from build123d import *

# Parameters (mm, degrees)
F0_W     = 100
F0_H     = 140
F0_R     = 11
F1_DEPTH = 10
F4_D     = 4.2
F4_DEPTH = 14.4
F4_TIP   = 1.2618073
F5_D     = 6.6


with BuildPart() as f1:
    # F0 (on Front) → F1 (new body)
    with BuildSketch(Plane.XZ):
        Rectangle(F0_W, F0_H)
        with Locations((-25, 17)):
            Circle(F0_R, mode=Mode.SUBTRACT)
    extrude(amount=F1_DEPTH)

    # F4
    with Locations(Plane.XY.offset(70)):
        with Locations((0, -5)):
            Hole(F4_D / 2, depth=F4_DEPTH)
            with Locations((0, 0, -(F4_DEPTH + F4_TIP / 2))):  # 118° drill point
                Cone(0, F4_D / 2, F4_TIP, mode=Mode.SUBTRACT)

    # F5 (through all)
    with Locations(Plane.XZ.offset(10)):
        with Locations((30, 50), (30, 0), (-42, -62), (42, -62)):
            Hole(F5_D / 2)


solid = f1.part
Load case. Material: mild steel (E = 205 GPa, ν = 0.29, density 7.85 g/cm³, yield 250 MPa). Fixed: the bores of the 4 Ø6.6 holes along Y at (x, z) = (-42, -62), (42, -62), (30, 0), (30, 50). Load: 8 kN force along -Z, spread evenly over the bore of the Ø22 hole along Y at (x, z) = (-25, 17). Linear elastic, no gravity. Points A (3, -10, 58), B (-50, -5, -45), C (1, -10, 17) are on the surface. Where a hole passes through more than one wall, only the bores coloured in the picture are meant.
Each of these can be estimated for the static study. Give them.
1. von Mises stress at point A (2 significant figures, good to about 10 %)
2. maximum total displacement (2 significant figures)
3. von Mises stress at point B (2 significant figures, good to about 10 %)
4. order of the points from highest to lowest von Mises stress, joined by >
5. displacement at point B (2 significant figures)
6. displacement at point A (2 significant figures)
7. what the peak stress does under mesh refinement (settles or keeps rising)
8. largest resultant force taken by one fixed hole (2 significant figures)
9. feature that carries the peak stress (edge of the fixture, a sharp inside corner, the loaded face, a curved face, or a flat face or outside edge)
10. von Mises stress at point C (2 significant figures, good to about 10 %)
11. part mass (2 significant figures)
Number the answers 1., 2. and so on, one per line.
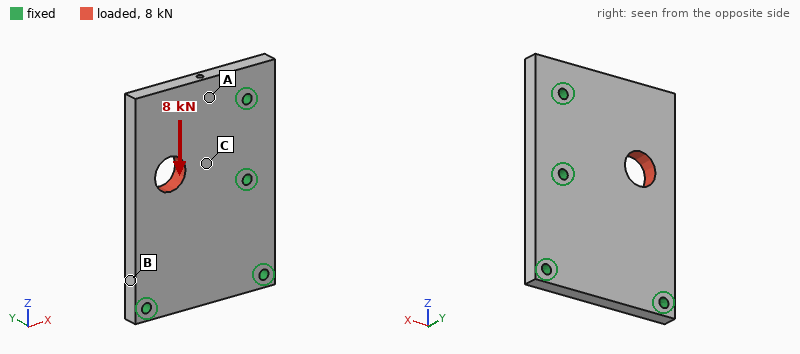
1. 5.5 MPa
2. 6.7 µm
3. 17 MPa
4. B > C > A
5. 1.2 µm
6. 2.7 µm
7. keeps rising
8. 3.2 kN
9. edge of the fixture
10. 11 MPa
11. 1.1 kg
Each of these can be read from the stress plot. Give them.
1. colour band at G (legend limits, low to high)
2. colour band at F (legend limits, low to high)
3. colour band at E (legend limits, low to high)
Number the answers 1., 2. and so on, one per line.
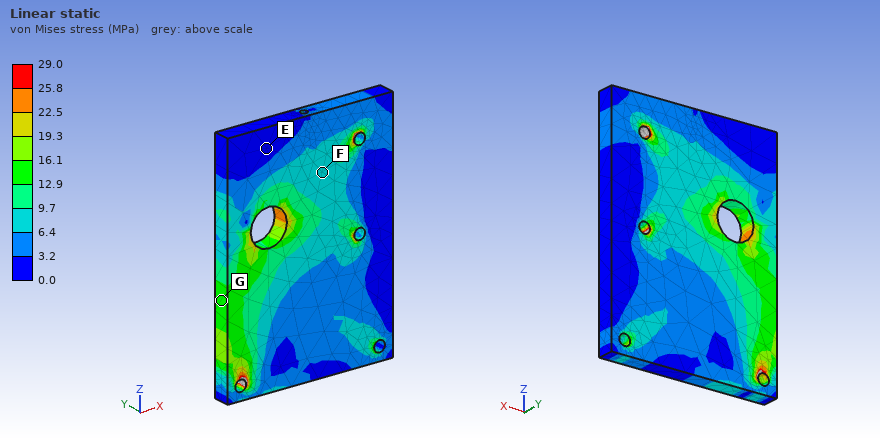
1. 12.9 to 16.1 MPa
2. 6.4 to 9.7 MPa
3. 0.0 to 3.2 MPa
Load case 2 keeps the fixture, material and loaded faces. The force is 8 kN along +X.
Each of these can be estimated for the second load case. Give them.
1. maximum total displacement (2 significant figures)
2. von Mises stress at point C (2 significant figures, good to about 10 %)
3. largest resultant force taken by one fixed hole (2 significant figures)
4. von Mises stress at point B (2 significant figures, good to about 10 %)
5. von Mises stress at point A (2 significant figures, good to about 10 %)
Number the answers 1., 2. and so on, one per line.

1. 5.6 µm
2. 11 MPa
3. 3.5 kN
4. 3.5 MPa
5. 6.6 MPa
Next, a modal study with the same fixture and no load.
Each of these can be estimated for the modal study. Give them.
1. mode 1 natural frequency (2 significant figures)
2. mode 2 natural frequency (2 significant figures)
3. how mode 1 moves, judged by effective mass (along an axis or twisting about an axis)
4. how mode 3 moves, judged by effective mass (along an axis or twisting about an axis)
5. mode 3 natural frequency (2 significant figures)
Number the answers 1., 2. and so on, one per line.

1. 1600 Hz
2. 3800 Hz
3. along Y
4. along Y
5. 6200 Hz
